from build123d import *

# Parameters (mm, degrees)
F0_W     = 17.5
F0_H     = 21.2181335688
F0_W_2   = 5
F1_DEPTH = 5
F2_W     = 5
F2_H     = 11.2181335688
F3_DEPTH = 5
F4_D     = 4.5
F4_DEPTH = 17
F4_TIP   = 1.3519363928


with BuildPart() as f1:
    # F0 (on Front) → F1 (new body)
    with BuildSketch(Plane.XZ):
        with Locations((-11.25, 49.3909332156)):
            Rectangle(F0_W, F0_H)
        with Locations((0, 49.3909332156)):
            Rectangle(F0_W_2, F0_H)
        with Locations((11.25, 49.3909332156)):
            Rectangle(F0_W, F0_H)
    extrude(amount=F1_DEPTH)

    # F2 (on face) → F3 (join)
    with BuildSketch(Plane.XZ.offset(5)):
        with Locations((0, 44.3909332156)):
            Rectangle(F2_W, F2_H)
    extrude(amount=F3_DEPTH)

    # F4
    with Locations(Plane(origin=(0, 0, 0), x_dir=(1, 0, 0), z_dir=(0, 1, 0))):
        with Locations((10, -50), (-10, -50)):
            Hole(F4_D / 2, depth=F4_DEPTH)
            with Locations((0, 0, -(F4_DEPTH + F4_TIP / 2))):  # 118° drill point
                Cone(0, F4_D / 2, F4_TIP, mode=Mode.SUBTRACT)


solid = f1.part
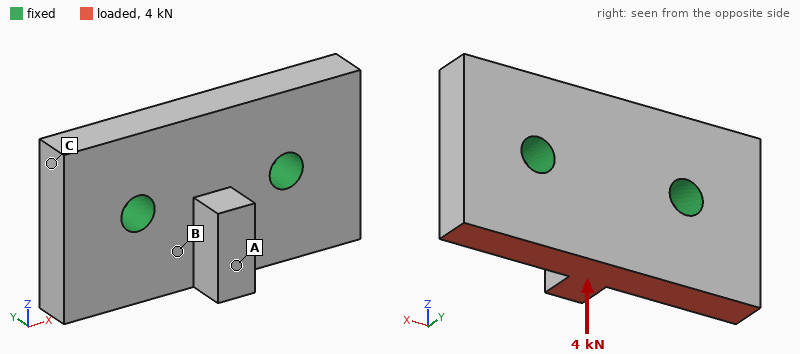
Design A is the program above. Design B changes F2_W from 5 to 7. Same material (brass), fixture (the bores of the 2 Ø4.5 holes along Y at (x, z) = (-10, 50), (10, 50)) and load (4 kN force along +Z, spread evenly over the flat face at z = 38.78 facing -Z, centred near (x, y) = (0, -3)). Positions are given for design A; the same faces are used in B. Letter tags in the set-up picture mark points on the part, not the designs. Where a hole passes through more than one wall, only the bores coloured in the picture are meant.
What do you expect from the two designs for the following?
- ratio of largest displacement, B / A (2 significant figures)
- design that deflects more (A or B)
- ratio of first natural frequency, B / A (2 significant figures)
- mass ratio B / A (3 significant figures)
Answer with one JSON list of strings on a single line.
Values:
["1.1", "B", "0.97", "1.03"]
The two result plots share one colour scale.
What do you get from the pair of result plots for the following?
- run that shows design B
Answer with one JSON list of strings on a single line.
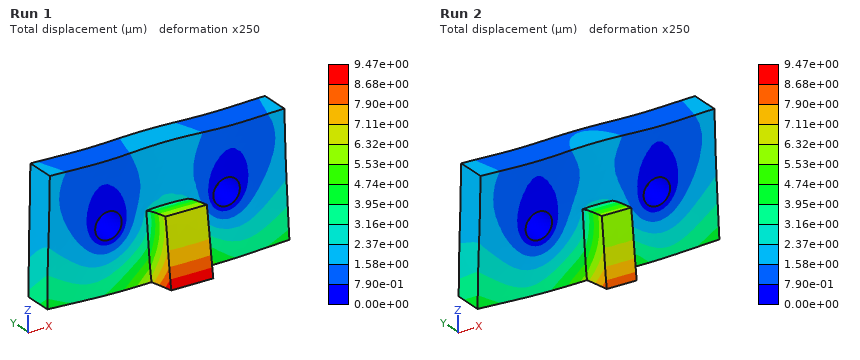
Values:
["Run 1"]
